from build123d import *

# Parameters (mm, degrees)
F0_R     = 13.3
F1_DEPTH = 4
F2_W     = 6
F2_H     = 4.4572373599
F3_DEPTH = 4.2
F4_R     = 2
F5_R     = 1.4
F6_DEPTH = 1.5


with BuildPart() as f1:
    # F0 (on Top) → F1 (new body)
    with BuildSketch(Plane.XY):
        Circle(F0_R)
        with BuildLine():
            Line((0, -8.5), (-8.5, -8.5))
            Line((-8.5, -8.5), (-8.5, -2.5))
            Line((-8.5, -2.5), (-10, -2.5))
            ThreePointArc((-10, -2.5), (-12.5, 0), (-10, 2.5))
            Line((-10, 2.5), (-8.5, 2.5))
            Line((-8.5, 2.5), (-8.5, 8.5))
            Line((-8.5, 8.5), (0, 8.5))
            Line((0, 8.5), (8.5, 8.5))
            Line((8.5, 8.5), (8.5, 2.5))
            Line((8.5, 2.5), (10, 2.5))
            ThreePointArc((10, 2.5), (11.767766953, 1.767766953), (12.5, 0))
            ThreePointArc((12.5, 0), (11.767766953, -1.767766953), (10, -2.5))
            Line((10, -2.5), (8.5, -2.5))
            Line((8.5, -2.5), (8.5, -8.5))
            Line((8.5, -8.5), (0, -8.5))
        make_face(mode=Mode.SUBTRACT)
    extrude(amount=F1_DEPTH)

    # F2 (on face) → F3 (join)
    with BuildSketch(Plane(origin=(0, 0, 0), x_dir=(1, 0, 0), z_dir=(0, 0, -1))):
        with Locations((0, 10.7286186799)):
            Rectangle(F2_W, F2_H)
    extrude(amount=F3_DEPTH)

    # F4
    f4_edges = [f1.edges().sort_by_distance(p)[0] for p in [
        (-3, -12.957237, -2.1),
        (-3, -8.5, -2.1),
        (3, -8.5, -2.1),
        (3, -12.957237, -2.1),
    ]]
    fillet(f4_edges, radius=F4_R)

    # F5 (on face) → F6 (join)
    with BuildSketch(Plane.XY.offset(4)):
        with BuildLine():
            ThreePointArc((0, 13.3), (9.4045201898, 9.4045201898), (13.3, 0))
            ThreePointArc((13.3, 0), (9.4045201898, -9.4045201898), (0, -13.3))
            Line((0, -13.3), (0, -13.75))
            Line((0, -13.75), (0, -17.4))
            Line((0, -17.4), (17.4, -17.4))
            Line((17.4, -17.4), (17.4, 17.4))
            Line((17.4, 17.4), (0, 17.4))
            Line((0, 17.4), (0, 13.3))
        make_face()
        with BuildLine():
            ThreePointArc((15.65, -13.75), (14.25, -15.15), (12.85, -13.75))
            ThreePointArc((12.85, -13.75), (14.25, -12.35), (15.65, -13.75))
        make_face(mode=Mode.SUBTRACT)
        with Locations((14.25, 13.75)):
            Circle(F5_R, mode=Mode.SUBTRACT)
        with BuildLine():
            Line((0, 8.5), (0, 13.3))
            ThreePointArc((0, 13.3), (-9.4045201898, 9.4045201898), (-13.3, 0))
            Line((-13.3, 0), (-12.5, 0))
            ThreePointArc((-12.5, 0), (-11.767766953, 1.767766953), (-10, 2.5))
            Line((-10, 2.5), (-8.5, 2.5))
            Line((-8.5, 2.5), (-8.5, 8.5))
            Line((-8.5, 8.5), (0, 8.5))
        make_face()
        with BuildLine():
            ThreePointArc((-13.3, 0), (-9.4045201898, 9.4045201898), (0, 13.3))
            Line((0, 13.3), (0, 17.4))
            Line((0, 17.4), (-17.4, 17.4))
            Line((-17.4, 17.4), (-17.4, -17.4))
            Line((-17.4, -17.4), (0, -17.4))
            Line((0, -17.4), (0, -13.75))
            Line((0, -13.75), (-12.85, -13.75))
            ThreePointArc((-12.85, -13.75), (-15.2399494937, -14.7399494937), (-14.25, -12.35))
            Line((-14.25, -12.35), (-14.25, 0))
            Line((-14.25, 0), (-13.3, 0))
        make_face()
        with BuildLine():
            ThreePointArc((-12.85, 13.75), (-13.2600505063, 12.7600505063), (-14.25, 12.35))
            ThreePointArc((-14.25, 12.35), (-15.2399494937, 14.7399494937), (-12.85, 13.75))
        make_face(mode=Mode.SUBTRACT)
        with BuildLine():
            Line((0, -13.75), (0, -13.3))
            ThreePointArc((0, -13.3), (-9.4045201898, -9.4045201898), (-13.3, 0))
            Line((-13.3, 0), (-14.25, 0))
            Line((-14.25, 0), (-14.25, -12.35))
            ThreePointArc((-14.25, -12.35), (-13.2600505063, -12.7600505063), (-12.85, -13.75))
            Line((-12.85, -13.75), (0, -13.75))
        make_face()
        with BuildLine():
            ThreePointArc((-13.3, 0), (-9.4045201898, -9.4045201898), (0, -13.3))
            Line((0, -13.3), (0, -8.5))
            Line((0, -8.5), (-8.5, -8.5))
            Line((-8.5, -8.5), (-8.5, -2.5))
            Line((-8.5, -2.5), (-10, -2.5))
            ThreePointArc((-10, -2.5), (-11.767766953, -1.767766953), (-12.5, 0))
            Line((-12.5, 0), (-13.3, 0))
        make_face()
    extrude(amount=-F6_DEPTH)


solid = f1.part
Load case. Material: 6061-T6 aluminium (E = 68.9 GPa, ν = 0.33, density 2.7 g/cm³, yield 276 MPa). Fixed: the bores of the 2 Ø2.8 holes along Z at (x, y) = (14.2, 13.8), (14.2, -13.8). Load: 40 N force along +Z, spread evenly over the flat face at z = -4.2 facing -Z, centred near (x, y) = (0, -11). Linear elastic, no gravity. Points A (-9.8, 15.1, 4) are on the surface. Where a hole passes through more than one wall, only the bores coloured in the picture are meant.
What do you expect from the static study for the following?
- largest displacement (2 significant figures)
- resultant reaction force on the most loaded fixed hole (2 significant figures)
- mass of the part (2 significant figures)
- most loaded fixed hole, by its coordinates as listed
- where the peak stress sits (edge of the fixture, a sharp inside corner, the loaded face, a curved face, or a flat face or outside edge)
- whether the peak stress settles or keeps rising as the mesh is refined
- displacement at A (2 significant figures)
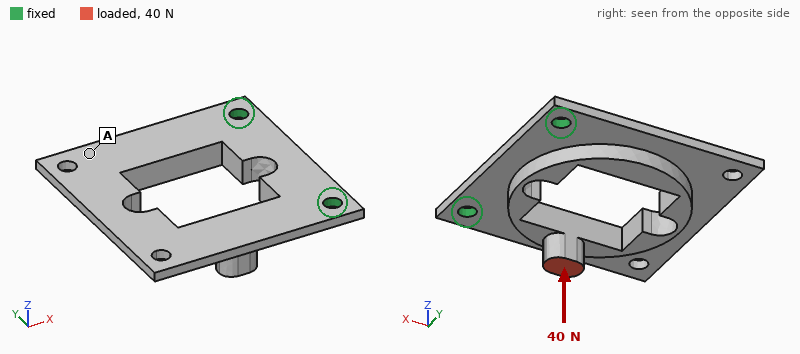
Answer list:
0.18 mm
37 N
5.3 g
(14.2, -13.8)
edge of the fixture
keeps rising
0.091 mm
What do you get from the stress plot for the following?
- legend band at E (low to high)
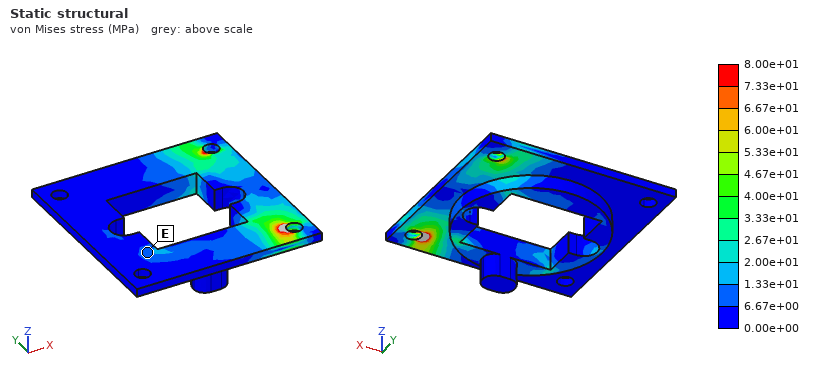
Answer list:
6.67e+00 to 1.33e+01 MPa
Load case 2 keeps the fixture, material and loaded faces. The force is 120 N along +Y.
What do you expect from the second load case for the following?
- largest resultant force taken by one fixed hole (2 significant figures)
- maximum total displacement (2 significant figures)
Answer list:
89 N
83 µm
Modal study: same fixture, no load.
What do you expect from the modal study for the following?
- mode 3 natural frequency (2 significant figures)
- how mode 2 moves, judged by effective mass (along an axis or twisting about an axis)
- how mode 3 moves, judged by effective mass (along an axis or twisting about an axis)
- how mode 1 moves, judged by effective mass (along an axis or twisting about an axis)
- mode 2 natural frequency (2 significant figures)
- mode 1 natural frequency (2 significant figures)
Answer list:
8200 Hz
twisting about X
along Y
along Z
3900 Hz
1300 Hz
